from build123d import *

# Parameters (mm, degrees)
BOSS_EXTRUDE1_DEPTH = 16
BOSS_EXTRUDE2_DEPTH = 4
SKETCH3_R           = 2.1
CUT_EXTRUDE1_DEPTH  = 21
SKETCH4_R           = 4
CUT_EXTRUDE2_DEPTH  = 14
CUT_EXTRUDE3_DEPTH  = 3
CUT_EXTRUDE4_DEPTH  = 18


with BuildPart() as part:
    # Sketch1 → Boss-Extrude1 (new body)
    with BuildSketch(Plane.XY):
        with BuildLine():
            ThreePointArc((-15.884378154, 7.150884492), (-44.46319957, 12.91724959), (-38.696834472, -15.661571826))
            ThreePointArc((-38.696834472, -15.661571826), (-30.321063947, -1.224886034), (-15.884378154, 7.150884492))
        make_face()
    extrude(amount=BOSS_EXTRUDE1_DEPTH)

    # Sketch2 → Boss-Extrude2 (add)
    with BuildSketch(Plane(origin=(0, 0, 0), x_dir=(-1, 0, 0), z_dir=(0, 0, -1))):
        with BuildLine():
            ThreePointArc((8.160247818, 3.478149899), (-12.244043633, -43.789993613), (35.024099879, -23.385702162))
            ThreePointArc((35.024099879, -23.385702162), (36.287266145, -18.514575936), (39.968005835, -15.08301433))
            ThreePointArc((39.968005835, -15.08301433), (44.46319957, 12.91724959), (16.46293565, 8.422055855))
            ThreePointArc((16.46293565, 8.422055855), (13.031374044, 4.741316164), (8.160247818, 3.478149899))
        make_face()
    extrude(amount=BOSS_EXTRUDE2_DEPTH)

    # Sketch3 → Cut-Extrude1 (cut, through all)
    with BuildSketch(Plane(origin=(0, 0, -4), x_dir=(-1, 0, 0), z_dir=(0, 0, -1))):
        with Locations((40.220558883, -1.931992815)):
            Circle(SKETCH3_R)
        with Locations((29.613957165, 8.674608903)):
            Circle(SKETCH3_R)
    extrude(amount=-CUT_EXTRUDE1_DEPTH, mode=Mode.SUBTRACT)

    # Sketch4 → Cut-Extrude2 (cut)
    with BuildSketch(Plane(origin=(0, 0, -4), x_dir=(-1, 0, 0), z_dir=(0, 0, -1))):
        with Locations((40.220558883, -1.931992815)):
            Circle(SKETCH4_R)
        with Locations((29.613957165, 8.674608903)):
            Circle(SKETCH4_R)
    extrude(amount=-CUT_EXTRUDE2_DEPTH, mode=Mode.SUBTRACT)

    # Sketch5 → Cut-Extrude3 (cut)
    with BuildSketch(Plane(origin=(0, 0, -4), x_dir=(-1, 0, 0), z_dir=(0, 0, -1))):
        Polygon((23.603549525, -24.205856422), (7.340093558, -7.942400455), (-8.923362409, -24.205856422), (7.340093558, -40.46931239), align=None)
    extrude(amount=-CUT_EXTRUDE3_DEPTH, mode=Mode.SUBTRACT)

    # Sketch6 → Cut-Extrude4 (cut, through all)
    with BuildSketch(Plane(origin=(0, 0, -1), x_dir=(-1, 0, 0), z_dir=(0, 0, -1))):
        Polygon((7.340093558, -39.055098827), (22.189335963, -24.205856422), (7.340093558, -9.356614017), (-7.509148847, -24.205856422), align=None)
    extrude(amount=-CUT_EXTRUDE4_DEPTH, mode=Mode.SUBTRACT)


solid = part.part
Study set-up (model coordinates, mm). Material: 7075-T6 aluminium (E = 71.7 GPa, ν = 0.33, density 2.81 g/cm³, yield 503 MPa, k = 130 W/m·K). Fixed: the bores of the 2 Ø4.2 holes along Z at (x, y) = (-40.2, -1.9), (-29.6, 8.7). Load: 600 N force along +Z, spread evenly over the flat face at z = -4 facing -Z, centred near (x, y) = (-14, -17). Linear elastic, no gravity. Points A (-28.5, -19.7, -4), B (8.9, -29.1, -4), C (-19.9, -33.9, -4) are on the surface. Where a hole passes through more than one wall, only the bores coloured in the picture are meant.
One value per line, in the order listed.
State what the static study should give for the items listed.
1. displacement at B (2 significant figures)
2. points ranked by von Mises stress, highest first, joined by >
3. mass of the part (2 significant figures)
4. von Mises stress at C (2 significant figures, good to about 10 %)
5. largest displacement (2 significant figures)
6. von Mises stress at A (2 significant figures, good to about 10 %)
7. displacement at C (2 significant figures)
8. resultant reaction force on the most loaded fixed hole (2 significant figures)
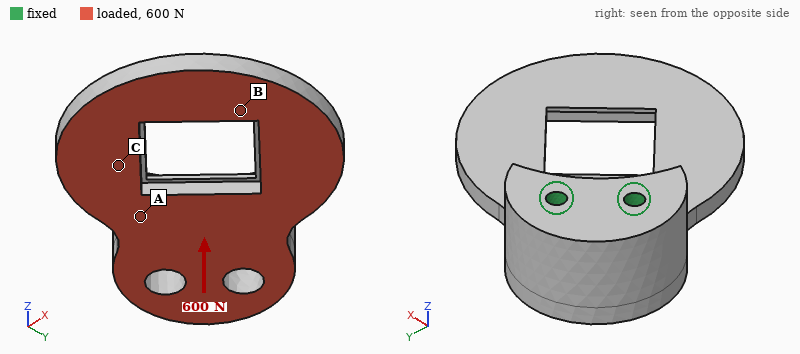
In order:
0.87 mm
A > C > B
54 g
45 MPa
1.2 mm
100 MPa
0.45 mm
300 N
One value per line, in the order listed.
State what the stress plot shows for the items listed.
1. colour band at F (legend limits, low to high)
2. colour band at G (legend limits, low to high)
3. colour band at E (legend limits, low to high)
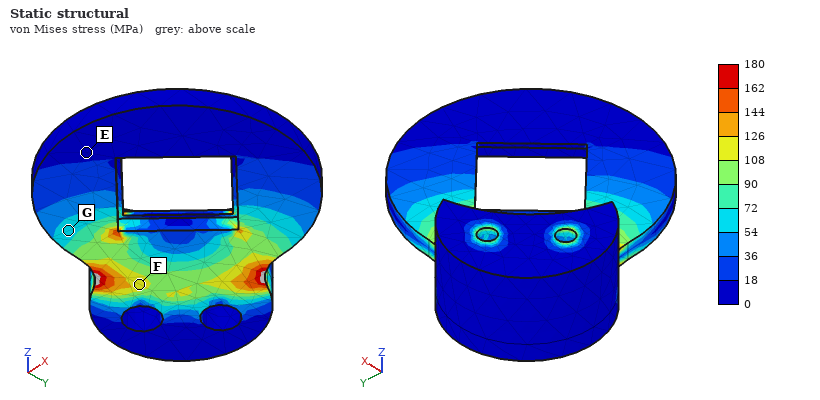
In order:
108 to 126 MPa
54 to 72 MPa
0 to 18 MPa
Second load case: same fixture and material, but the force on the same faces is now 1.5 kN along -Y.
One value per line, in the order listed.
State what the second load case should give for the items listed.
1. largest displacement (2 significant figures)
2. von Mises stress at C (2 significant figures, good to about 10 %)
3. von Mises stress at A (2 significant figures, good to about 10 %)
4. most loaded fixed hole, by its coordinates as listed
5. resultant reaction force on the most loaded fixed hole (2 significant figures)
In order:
0.30 mm
19 MPa
34 MPa
(-29.6, 8.7)
2.4 kN
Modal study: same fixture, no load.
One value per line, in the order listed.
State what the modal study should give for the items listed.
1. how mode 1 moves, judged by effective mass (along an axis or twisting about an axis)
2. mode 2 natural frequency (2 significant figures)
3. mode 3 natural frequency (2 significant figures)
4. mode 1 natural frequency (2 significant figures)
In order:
along Z
2100 Hz
3100 Hz
830 Hz
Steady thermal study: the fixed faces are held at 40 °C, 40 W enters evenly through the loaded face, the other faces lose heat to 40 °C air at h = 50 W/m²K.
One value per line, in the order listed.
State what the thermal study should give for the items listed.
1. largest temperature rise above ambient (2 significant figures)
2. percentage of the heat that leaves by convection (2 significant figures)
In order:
61 K
21 %
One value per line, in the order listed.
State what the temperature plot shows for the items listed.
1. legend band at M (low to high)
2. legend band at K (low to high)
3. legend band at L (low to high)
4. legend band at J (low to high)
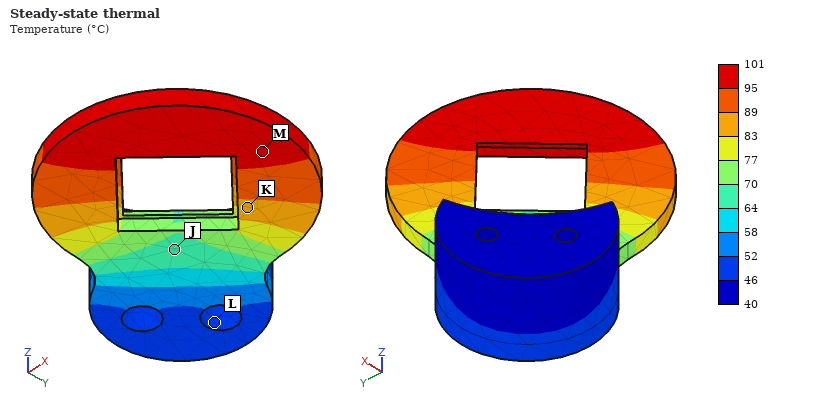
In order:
95 to 101 °C
83 to 89 °C
46 to 52 °C
64 to 70 °C
